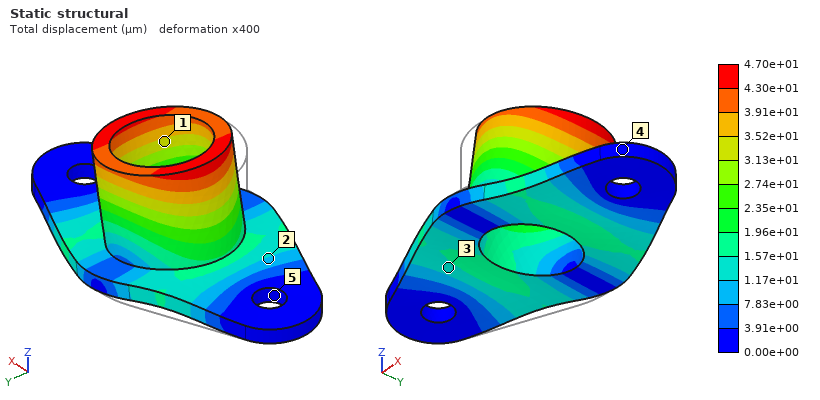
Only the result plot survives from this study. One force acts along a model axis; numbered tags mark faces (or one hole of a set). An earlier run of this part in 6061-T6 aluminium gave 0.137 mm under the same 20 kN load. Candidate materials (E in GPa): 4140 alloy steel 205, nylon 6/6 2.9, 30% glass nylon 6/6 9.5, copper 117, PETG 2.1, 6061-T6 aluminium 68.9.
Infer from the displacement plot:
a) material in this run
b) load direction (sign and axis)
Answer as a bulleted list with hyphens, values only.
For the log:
- 4140 alloy steel
- +X
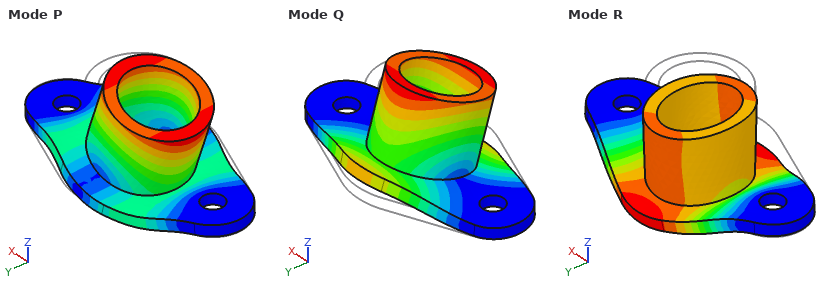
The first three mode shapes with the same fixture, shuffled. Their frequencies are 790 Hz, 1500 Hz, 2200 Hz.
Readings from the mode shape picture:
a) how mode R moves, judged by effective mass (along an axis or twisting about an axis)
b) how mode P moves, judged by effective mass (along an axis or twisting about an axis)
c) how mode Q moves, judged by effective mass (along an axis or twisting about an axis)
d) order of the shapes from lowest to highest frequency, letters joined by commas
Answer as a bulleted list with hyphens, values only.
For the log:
- along Z
- along X
- along Y
- Q, R, P
